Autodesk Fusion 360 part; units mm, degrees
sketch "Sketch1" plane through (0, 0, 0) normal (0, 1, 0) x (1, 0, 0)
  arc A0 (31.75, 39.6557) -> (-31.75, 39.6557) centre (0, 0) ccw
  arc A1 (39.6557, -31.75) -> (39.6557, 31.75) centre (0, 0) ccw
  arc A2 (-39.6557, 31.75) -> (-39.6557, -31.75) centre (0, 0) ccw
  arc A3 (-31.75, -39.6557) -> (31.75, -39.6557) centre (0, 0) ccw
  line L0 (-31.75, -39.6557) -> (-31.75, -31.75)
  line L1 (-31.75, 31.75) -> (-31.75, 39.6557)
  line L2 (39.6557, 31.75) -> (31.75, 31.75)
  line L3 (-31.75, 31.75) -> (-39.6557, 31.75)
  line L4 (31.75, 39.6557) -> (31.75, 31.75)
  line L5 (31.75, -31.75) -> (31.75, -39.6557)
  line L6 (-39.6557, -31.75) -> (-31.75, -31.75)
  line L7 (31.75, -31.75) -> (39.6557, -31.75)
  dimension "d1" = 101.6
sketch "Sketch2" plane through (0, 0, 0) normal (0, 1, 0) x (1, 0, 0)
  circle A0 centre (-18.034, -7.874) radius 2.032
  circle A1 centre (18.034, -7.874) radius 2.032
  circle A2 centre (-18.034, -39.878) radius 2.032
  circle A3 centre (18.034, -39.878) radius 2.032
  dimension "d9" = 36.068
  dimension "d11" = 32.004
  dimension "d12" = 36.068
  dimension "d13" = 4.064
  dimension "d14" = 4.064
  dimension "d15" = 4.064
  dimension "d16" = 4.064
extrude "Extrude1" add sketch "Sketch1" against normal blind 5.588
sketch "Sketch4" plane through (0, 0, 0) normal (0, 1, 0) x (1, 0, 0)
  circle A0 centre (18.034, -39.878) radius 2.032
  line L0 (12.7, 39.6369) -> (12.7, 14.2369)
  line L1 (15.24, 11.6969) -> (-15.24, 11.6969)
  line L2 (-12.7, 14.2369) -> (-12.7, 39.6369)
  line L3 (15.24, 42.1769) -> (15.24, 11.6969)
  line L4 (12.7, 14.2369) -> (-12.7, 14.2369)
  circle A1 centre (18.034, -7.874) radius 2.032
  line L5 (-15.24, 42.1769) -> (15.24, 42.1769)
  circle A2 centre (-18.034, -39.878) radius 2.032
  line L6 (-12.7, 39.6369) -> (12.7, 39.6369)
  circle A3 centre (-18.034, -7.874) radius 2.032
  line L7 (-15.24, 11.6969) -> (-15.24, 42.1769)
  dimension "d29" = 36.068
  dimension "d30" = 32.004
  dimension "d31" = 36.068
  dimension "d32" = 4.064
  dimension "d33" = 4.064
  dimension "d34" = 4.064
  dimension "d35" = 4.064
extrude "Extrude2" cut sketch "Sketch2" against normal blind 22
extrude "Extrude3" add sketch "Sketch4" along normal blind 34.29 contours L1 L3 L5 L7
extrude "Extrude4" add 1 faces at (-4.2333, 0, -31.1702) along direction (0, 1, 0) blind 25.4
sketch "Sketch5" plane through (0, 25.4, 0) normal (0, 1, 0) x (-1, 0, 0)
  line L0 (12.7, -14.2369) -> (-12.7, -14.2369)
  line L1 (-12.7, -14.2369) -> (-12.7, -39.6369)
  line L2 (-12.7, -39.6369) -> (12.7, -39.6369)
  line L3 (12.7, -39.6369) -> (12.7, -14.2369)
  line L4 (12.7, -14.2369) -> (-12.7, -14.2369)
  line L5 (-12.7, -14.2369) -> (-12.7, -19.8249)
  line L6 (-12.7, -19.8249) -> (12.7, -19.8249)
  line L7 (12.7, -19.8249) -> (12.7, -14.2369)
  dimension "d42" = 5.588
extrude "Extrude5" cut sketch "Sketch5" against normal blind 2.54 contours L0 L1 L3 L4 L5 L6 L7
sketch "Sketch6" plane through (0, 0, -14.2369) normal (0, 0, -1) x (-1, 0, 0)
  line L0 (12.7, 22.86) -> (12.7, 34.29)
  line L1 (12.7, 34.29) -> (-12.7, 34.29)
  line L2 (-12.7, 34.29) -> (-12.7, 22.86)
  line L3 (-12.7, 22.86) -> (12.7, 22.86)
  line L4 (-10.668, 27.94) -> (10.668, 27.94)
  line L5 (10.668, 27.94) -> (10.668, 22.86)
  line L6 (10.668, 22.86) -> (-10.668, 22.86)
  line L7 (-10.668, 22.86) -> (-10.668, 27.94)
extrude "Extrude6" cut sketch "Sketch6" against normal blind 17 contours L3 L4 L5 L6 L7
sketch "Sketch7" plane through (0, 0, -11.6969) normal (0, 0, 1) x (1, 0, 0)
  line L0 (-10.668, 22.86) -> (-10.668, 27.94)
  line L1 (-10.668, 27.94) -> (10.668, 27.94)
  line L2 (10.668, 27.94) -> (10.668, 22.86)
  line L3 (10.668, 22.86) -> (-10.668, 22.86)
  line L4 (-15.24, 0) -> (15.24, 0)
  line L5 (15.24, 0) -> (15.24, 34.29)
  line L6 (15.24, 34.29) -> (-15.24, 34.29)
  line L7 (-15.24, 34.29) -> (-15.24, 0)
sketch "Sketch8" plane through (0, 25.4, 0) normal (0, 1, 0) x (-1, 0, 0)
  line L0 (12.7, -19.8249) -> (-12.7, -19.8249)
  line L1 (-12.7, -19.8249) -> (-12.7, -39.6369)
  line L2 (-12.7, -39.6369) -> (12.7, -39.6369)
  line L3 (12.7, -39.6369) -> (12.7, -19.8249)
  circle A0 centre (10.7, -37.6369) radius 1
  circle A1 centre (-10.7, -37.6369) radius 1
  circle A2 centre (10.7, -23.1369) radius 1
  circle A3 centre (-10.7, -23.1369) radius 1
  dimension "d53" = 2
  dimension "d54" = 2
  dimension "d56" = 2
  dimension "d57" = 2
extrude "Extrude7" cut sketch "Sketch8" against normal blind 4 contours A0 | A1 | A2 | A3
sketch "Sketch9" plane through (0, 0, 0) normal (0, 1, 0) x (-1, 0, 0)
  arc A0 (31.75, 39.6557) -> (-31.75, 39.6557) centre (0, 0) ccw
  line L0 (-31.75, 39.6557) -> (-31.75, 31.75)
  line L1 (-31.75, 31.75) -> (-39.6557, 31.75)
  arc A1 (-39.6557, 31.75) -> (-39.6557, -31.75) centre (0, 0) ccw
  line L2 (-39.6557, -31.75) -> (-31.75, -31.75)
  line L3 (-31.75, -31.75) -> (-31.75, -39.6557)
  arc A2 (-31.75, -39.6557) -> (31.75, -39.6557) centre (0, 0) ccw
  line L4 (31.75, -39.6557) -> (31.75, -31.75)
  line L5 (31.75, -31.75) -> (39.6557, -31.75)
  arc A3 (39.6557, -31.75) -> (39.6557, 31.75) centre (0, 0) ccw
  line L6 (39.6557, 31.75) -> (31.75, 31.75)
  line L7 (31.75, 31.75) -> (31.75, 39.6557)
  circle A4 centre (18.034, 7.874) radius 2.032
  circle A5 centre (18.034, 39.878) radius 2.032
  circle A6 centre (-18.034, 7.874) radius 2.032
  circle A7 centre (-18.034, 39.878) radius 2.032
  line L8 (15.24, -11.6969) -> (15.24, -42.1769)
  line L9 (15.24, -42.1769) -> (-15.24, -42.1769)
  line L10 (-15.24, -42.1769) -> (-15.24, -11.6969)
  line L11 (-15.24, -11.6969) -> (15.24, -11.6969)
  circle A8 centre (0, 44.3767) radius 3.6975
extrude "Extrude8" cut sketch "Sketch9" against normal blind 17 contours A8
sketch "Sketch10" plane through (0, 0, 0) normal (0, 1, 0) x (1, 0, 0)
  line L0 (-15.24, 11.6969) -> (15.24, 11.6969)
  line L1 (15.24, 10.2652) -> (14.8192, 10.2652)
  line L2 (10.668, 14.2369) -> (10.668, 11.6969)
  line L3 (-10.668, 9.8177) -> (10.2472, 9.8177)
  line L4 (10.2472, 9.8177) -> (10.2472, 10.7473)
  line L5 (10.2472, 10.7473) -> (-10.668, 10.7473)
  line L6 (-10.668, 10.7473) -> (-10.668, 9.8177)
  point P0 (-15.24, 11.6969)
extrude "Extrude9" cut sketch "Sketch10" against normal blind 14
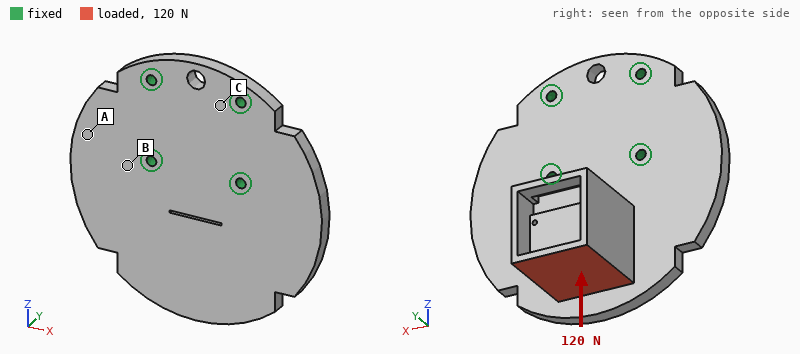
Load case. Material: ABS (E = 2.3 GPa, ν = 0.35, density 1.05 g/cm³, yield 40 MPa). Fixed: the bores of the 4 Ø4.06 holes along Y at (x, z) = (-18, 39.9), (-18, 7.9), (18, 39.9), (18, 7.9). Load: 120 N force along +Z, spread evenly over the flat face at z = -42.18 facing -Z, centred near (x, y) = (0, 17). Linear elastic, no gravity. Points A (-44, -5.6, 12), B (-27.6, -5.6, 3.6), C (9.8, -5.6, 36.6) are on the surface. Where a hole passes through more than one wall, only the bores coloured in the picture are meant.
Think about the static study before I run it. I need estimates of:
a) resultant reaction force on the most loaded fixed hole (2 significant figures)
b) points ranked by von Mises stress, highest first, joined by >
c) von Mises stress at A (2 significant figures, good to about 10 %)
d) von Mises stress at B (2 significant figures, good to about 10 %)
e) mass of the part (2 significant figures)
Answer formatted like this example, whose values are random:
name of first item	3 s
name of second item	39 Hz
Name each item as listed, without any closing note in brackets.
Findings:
resultant reaction force on the most loaded fixed hole	55 N
points ranked by von Mises stress, highest first, joined by >	B > A > C
von Mises stress at A	2.4 MPa
von Mises stress at B	4.2 MPa
mass of the part	73 g
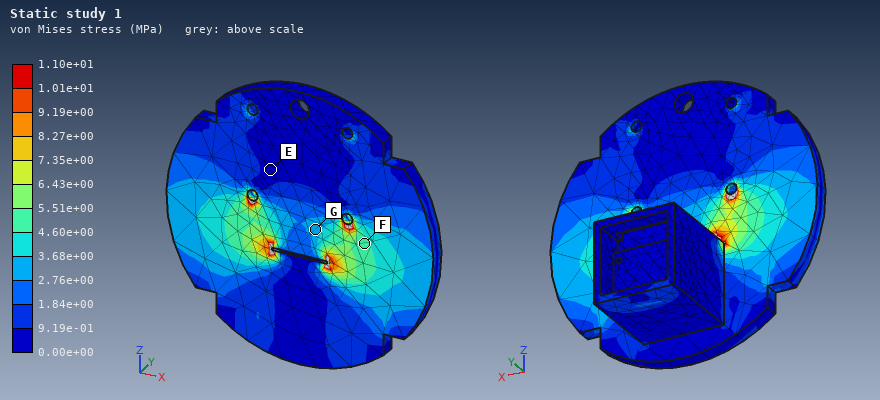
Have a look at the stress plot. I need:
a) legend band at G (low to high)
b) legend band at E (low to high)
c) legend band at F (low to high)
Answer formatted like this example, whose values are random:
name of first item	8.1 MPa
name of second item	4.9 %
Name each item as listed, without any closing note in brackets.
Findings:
legend band at G	2.76e+00 to 3.68e+00 MPa
legend band at E	0.00e+00 to 9.19e-01 MPa
legend band at F	4.60e+00 to 5.51e+00 MPa
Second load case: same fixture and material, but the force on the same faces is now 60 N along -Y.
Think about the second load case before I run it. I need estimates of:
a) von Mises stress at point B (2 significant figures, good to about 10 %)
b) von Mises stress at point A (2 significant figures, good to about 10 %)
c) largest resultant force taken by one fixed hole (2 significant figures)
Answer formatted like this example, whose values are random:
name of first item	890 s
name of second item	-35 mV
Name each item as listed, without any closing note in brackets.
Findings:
von Mises stress at point B	4.7 MPa
von Mises stress at point A	2.6 MPa
largest resultant force taken by one fixed hole	53 N
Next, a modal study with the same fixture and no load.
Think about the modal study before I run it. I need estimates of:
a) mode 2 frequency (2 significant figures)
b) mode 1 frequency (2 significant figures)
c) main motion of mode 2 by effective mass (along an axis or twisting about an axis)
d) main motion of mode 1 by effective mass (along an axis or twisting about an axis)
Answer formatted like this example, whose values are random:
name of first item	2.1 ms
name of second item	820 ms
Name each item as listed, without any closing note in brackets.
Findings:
mode 2 frequency	710 Hz
mode 1 frequency	250 Hz
main motion of mode 2 by effective mass	along X
main motion of mode 1 by effective mass	along Y
